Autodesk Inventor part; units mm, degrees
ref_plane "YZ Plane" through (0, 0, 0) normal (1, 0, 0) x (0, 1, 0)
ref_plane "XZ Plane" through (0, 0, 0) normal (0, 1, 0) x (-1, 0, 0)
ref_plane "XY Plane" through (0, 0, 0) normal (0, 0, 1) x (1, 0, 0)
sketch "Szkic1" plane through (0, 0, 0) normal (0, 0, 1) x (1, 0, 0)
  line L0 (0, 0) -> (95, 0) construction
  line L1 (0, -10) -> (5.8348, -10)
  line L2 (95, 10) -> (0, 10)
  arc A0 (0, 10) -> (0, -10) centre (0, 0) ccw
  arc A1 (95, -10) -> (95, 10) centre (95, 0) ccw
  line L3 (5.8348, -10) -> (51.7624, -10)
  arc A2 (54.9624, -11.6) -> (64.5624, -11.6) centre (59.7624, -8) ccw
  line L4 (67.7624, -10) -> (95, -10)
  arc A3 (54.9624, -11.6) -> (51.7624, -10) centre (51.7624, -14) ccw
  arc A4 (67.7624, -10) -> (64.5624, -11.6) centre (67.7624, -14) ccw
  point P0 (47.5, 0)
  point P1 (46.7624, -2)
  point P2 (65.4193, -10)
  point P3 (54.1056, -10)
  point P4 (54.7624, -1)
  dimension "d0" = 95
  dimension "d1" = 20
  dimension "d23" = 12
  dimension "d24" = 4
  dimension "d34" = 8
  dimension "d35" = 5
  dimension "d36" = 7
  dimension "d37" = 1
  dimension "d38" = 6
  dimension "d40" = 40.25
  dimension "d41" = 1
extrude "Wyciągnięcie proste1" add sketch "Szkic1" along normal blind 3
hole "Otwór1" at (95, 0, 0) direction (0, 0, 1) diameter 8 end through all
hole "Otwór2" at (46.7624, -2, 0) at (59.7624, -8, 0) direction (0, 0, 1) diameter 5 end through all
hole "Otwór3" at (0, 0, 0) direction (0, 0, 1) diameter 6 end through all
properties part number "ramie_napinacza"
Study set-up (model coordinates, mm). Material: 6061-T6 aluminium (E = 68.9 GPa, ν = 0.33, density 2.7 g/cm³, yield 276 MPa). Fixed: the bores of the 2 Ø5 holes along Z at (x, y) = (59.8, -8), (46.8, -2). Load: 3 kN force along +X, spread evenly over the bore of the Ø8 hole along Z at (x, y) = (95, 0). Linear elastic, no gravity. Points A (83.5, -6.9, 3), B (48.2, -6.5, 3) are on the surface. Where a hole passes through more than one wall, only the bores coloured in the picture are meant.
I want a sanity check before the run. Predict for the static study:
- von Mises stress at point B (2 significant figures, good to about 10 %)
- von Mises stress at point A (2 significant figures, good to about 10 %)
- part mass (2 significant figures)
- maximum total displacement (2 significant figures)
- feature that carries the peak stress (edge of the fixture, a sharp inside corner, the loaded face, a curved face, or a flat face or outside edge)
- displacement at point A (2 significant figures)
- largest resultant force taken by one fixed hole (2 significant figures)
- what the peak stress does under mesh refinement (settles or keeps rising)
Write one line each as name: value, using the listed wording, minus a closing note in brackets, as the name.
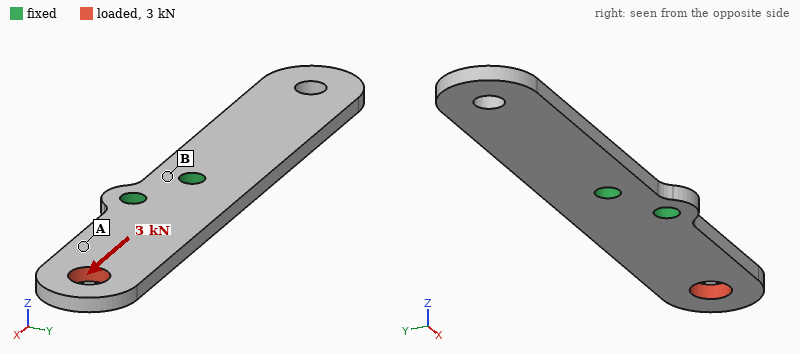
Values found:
von Mises stress at point B: 15 MPa
von Mises stress at point A: 52 MPa
part mass: 17 g
maximum total displacement: 62 µm
feature that carries the peak stress: edge of the fixture
displacement at point A: 29 µm
largest resultant force taken by one fixed hole: 1.7 kN
what the peak stress does under mesh refinement: keeps rising
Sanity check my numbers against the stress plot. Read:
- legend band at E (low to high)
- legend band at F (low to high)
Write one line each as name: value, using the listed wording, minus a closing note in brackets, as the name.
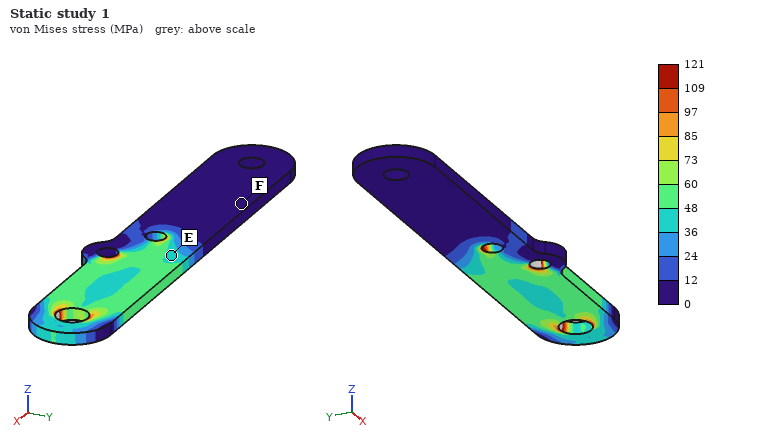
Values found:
legend band at E: 36 to 48 MPa
legend band at F: 0 to 12 MPa
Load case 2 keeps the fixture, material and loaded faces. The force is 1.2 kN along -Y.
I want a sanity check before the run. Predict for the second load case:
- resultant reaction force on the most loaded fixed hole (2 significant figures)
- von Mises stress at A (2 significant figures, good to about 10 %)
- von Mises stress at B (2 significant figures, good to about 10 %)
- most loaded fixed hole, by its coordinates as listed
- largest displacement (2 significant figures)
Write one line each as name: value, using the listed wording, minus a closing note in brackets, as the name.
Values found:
resultant reaction force on the most loaded fixed hole: 3.3 kN
von Mises stress at A: 51 MPa
von Mises stress at B: 23 MPa
most loaded fixed hole, by its coordinates as listed: (59.8, -8)
largest displacement: 0.27 mm
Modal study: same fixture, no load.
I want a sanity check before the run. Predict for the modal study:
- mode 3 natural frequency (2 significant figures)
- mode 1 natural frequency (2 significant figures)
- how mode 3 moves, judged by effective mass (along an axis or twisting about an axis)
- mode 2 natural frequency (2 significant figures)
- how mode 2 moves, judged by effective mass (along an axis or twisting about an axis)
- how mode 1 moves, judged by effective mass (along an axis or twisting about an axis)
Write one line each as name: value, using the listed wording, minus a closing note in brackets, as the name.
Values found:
mode 3 natural frequency: 4200 Hz
mode 1 natural frequency: 880 Hz
how mode 3 moves, judged by effective mass: along Y
mode 2 natural frequency: 1400 Hz
how mode 2 moves, judged by effective mass: along Z
how mode 1 moves, judged by effective mass: along Z
